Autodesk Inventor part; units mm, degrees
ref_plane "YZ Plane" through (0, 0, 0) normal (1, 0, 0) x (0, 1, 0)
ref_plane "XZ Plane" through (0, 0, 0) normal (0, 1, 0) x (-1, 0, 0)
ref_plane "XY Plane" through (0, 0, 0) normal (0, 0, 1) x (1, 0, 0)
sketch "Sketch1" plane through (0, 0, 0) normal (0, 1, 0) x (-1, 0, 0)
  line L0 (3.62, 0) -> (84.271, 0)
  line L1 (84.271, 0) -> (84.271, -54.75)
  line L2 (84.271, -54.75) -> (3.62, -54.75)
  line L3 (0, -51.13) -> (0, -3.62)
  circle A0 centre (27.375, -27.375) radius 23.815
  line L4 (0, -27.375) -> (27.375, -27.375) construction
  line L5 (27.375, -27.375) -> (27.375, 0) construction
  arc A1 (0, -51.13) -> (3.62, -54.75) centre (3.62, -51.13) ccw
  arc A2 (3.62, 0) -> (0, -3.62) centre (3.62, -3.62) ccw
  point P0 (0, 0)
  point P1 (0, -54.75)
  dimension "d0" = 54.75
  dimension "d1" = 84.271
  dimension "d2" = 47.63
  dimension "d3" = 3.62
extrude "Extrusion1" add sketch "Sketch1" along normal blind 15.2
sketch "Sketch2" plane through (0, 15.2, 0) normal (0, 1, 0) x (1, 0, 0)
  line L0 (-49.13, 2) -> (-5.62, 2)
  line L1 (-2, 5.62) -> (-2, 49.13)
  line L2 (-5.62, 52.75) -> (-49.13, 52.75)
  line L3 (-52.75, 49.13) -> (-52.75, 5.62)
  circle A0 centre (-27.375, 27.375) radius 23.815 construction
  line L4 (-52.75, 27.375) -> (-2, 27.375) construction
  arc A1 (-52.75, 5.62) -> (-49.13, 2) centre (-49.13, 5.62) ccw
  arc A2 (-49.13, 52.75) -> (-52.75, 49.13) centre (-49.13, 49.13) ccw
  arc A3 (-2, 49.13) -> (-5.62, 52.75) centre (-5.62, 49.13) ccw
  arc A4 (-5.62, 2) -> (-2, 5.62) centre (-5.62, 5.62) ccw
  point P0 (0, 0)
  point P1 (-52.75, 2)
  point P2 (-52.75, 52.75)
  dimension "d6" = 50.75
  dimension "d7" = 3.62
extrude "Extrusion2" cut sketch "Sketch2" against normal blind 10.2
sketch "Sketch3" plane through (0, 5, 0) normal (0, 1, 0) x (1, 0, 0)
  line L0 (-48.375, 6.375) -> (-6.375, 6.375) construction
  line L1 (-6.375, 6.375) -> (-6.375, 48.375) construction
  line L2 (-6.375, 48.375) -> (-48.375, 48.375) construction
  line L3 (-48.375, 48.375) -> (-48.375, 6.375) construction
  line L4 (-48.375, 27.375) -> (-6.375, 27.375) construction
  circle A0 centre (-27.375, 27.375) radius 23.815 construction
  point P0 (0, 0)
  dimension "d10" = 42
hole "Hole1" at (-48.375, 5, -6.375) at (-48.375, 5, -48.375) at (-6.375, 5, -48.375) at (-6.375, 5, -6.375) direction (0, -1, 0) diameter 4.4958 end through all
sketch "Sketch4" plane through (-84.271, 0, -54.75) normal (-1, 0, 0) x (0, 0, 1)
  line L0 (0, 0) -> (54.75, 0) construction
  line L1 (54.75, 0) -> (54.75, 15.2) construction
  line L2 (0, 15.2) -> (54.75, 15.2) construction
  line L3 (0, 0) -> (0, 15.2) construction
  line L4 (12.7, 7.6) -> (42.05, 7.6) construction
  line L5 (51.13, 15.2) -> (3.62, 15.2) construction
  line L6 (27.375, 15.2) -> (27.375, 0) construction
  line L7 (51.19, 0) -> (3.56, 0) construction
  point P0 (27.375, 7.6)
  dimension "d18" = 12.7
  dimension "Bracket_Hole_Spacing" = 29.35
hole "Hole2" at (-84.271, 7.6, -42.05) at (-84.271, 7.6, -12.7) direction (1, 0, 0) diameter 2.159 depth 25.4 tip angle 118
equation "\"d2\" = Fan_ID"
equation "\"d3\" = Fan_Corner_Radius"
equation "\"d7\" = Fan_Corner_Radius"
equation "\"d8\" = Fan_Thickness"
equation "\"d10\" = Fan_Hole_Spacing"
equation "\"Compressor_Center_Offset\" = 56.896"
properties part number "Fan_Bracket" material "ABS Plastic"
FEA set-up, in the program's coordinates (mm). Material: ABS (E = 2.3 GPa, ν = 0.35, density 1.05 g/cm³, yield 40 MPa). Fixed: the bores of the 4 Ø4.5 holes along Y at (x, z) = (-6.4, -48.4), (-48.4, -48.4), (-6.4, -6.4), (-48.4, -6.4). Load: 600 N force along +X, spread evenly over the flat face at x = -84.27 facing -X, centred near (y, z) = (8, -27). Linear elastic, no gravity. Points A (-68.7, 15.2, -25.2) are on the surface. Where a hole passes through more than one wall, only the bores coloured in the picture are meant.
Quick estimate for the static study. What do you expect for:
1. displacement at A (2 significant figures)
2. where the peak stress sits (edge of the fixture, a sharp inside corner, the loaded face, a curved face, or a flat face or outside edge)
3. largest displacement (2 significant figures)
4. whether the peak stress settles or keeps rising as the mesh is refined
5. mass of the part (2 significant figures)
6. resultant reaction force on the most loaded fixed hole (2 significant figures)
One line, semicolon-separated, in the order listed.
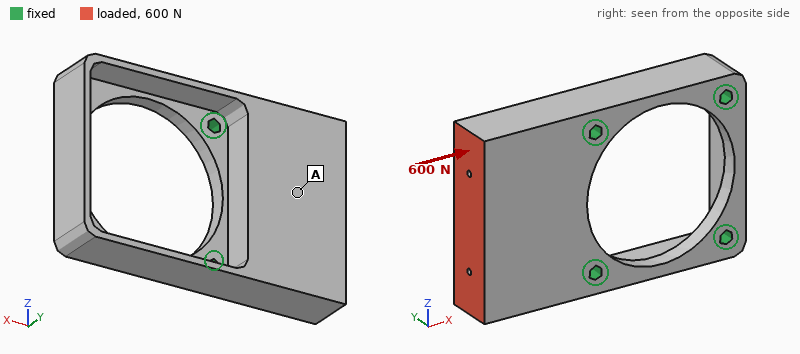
0.17 mm; edge of the fixture; 0.27 mm; keeps rising; 36 g; 270 N
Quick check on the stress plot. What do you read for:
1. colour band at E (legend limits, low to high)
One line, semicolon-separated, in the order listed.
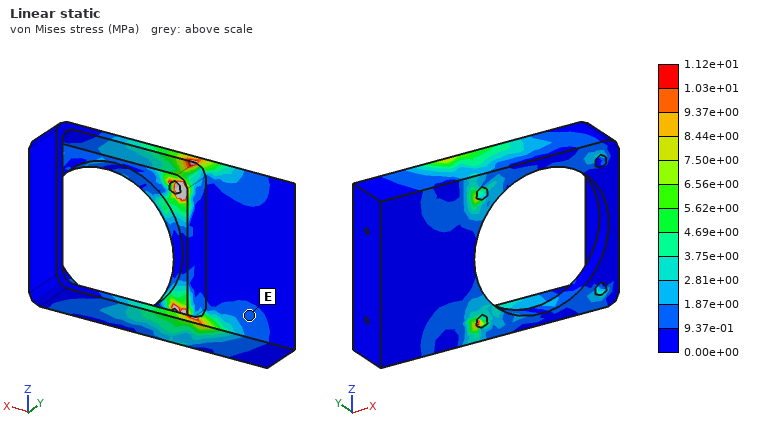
9.37e-01 to 1.87e+00 MPa
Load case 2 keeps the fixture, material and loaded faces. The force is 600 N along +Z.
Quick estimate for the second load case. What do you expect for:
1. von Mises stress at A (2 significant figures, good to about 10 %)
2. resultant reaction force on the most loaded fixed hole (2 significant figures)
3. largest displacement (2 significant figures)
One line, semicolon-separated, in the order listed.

1.2 MPa; 530 N; 0.13 mm
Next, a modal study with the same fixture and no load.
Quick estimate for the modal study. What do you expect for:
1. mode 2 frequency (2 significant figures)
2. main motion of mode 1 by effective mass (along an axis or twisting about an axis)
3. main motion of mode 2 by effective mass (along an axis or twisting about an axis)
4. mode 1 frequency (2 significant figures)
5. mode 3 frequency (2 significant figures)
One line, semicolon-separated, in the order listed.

2700 Hz; along Y; twisting about X; 850 Hz; 3200 Hz
